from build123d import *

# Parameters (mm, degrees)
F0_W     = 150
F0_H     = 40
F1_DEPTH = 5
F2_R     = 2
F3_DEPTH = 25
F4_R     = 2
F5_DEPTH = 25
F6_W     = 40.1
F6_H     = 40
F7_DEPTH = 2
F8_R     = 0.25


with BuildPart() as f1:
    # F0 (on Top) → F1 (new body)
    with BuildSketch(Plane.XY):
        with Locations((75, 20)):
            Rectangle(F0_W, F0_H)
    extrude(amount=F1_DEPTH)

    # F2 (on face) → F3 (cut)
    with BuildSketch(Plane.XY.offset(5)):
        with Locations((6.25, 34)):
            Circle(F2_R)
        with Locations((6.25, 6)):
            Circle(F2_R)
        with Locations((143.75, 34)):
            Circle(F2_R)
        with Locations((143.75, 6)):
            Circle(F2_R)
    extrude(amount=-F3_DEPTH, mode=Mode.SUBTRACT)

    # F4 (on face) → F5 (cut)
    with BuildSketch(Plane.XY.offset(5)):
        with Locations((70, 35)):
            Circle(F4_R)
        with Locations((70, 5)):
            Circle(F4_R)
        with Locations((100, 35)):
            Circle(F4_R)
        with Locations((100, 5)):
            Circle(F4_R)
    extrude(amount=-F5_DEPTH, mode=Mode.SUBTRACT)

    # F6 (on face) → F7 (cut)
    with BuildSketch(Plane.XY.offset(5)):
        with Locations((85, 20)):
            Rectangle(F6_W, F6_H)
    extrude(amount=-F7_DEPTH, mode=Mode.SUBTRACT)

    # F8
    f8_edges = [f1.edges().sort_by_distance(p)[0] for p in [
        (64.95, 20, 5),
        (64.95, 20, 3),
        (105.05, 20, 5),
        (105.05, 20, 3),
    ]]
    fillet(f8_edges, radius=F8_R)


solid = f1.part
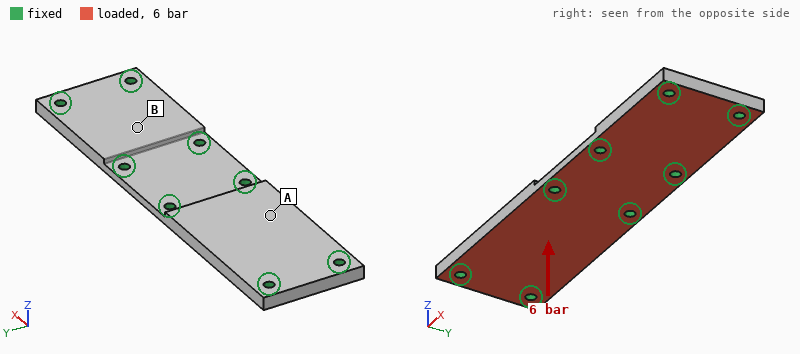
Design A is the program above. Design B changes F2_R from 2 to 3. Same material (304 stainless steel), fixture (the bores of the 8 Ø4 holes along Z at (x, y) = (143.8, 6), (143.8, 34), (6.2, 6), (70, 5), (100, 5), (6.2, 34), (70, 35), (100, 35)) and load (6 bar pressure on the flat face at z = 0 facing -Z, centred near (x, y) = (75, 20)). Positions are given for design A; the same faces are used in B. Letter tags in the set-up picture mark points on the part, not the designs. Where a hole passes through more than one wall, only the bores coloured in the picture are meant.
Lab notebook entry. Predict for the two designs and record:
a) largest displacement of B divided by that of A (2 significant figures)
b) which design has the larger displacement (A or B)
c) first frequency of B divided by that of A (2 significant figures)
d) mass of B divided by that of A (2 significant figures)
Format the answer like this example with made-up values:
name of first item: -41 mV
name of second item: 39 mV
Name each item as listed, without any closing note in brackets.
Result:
largest displacement of B divided by that of A: 0.91
which design has the larger displacement: A
first frequency of B divided by that of A: 1.0
mass of B divided by that of A: 0.99
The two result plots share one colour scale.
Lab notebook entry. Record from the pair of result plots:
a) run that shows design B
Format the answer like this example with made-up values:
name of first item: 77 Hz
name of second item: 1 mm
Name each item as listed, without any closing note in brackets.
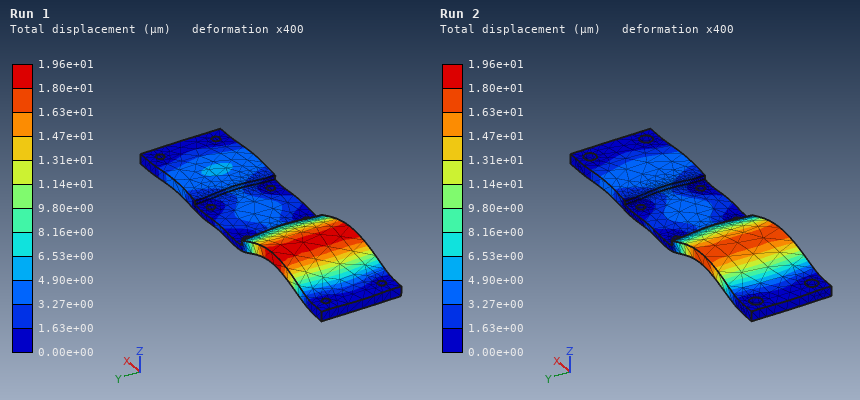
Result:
run that shows design B: Run 2
